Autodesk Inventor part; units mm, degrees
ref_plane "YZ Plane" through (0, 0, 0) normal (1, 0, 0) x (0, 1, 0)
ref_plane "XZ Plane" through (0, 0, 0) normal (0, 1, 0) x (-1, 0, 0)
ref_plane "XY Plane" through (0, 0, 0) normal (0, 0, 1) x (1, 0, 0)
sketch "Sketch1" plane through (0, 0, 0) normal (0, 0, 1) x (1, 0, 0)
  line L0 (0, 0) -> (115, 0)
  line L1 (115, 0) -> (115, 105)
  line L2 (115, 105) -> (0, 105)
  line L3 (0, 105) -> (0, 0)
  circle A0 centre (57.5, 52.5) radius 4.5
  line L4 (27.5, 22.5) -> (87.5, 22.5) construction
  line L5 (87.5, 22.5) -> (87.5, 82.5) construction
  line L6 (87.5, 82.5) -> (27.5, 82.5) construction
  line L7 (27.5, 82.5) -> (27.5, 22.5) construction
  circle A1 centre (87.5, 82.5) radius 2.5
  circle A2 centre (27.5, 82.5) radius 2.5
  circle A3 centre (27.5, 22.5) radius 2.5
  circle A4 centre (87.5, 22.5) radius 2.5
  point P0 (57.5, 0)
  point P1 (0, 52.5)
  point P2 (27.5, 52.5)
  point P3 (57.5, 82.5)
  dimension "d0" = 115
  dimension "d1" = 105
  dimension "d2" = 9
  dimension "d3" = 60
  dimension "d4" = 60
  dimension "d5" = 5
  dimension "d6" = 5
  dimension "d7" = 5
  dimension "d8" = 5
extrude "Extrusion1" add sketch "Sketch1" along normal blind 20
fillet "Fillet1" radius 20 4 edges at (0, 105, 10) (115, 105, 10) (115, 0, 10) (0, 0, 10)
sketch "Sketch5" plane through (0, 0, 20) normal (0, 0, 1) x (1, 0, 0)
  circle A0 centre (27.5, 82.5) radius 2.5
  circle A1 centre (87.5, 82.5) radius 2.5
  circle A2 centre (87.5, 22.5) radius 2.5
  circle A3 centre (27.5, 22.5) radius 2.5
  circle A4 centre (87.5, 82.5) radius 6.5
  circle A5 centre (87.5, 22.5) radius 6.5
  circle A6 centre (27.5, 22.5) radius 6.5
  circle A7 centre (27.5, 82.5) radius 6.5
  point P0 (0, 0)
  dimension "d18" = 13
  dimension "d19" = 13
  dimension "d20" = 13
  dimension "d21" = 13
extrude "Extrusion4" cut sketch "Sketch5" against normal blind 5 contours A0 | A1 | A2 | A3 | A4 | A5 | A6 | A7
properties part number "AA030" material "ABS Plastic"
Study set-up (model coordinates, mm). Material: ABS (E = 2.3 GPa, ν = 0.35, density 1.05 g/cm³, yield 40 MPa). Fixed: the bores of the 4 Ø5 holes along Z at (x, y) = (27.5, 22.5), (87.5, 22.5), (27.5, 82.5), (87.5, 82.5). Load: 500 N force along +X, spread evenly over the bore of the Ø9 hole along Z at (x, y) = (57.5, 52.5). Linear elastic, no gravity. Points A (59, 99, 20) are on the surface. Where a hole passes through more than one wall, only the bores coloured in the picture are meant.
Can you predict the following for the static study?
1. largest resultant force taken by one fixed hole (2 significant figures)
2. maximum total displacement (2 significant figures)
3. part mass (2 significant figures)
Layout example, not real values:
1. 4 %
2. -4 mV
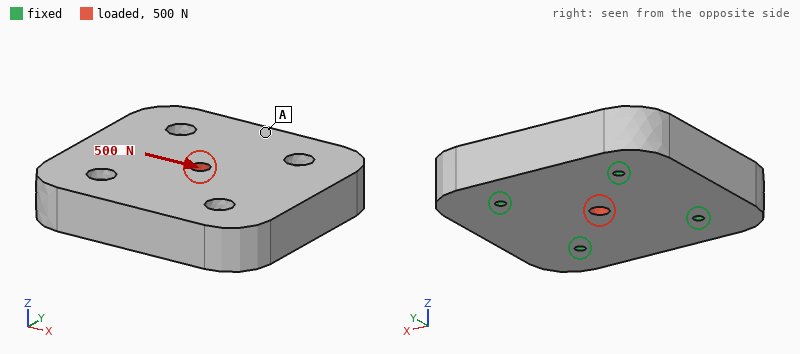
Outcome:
1. 130 N
2. 9.1 µm
3. 240 g
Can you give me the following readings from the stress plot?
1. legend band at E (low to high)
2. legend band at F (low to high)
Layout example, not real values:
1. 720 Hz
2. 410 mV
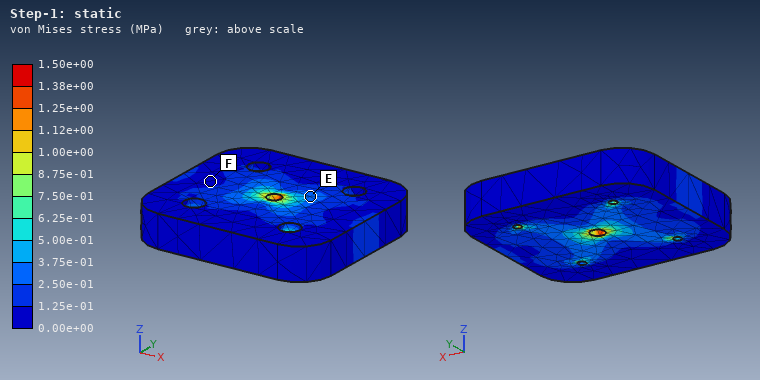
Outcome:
1. 2.50e-01 to 3.75e-01 MPa
2. 0.00e+00 to 1.25e-01 MPa
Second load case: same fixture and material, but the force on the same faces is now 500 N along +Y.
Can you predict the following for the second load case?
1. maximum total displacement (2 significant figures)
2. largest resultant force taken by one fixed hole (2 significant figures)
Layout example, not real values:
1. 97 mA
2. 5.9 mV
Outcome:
1. 9.2 µm
2. 130 N
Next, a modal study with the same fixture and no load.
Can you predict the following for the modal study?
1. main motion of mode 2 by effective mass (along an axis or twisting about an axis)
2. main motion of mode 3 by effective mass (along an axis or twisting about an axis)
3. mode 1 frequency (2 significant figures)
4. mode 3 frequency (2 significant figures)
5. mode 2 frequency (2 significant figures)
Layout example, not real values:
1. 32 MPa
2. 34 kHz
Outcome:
1. twisting about Y
2. along Z
3. 2700 Hz
4. 3400 Hz
5. 2900 Hz
